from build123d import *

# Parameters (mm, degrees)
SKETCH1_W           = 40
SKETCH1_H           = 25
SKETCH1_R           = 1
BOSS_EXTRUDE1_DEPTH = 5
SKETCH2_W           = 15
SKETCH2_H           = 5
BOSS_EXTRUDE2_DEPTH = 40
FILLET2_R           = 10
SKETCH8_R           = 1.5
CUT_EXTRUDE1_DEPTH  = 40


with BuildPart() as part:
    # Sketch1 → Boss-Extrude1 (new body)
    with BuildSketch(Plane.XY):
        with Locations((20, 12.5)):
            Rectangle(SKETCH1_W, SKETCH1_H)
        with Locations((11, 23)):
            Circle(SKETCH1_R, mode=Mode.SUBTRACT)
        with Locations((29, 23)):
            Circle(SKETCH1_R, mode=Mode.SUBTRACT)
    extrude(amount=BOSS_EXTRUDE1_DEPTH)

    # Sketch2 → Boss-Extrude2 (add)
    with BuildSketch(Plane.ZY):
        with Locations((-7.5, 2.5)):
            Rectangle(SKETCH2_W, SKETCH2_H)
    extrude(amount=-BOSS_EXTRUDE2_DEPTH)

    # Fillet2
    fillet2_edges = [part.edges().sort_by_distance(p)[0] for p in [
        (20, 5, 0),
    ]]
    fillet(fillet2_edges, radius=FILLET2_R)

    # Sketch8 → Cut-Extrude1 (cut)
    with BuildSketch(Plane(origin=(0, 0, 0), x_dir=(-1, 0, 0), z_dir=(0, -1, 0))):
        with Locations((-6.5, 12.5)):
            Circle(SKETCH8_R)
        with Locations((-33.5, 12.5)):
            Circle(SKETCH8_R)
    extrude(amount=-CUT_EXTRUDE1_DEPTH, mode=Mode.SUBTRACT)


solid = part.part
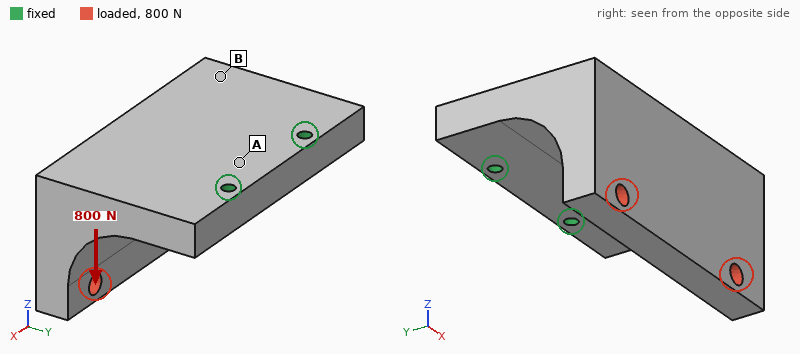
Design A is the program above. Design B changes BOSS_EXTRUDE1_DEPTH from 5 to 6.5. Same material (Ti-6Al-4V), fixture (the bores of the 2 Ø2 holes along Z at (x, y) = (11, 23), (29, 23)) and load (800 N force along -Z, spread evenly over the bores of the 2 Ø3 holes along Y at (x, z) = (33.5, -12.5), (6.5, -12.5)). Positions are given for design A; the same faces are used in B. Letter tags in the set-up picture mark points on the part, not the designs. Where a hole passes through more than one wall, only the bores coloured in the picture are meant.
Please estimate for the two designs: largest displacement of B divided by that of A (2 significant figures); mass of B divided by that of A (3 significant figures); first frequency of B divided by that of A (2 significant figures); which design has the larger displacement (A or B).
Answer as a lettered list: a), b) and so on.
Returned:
a) 0.52
b) 1.17
c) 1.3
d) A
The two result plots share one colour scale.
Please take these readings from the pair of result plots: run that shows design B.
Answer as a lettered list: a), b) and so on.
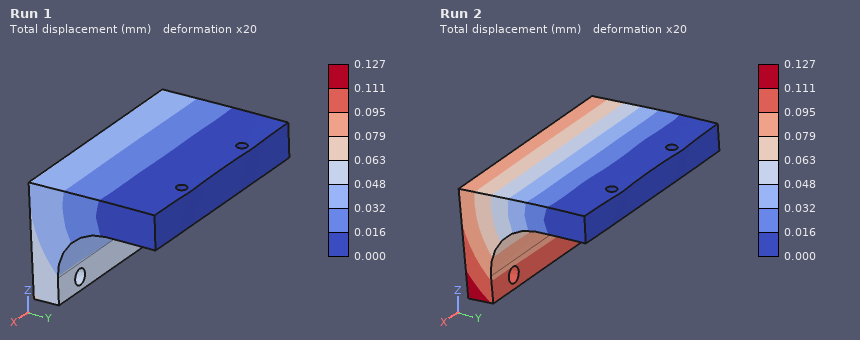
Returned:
a) Run 1
